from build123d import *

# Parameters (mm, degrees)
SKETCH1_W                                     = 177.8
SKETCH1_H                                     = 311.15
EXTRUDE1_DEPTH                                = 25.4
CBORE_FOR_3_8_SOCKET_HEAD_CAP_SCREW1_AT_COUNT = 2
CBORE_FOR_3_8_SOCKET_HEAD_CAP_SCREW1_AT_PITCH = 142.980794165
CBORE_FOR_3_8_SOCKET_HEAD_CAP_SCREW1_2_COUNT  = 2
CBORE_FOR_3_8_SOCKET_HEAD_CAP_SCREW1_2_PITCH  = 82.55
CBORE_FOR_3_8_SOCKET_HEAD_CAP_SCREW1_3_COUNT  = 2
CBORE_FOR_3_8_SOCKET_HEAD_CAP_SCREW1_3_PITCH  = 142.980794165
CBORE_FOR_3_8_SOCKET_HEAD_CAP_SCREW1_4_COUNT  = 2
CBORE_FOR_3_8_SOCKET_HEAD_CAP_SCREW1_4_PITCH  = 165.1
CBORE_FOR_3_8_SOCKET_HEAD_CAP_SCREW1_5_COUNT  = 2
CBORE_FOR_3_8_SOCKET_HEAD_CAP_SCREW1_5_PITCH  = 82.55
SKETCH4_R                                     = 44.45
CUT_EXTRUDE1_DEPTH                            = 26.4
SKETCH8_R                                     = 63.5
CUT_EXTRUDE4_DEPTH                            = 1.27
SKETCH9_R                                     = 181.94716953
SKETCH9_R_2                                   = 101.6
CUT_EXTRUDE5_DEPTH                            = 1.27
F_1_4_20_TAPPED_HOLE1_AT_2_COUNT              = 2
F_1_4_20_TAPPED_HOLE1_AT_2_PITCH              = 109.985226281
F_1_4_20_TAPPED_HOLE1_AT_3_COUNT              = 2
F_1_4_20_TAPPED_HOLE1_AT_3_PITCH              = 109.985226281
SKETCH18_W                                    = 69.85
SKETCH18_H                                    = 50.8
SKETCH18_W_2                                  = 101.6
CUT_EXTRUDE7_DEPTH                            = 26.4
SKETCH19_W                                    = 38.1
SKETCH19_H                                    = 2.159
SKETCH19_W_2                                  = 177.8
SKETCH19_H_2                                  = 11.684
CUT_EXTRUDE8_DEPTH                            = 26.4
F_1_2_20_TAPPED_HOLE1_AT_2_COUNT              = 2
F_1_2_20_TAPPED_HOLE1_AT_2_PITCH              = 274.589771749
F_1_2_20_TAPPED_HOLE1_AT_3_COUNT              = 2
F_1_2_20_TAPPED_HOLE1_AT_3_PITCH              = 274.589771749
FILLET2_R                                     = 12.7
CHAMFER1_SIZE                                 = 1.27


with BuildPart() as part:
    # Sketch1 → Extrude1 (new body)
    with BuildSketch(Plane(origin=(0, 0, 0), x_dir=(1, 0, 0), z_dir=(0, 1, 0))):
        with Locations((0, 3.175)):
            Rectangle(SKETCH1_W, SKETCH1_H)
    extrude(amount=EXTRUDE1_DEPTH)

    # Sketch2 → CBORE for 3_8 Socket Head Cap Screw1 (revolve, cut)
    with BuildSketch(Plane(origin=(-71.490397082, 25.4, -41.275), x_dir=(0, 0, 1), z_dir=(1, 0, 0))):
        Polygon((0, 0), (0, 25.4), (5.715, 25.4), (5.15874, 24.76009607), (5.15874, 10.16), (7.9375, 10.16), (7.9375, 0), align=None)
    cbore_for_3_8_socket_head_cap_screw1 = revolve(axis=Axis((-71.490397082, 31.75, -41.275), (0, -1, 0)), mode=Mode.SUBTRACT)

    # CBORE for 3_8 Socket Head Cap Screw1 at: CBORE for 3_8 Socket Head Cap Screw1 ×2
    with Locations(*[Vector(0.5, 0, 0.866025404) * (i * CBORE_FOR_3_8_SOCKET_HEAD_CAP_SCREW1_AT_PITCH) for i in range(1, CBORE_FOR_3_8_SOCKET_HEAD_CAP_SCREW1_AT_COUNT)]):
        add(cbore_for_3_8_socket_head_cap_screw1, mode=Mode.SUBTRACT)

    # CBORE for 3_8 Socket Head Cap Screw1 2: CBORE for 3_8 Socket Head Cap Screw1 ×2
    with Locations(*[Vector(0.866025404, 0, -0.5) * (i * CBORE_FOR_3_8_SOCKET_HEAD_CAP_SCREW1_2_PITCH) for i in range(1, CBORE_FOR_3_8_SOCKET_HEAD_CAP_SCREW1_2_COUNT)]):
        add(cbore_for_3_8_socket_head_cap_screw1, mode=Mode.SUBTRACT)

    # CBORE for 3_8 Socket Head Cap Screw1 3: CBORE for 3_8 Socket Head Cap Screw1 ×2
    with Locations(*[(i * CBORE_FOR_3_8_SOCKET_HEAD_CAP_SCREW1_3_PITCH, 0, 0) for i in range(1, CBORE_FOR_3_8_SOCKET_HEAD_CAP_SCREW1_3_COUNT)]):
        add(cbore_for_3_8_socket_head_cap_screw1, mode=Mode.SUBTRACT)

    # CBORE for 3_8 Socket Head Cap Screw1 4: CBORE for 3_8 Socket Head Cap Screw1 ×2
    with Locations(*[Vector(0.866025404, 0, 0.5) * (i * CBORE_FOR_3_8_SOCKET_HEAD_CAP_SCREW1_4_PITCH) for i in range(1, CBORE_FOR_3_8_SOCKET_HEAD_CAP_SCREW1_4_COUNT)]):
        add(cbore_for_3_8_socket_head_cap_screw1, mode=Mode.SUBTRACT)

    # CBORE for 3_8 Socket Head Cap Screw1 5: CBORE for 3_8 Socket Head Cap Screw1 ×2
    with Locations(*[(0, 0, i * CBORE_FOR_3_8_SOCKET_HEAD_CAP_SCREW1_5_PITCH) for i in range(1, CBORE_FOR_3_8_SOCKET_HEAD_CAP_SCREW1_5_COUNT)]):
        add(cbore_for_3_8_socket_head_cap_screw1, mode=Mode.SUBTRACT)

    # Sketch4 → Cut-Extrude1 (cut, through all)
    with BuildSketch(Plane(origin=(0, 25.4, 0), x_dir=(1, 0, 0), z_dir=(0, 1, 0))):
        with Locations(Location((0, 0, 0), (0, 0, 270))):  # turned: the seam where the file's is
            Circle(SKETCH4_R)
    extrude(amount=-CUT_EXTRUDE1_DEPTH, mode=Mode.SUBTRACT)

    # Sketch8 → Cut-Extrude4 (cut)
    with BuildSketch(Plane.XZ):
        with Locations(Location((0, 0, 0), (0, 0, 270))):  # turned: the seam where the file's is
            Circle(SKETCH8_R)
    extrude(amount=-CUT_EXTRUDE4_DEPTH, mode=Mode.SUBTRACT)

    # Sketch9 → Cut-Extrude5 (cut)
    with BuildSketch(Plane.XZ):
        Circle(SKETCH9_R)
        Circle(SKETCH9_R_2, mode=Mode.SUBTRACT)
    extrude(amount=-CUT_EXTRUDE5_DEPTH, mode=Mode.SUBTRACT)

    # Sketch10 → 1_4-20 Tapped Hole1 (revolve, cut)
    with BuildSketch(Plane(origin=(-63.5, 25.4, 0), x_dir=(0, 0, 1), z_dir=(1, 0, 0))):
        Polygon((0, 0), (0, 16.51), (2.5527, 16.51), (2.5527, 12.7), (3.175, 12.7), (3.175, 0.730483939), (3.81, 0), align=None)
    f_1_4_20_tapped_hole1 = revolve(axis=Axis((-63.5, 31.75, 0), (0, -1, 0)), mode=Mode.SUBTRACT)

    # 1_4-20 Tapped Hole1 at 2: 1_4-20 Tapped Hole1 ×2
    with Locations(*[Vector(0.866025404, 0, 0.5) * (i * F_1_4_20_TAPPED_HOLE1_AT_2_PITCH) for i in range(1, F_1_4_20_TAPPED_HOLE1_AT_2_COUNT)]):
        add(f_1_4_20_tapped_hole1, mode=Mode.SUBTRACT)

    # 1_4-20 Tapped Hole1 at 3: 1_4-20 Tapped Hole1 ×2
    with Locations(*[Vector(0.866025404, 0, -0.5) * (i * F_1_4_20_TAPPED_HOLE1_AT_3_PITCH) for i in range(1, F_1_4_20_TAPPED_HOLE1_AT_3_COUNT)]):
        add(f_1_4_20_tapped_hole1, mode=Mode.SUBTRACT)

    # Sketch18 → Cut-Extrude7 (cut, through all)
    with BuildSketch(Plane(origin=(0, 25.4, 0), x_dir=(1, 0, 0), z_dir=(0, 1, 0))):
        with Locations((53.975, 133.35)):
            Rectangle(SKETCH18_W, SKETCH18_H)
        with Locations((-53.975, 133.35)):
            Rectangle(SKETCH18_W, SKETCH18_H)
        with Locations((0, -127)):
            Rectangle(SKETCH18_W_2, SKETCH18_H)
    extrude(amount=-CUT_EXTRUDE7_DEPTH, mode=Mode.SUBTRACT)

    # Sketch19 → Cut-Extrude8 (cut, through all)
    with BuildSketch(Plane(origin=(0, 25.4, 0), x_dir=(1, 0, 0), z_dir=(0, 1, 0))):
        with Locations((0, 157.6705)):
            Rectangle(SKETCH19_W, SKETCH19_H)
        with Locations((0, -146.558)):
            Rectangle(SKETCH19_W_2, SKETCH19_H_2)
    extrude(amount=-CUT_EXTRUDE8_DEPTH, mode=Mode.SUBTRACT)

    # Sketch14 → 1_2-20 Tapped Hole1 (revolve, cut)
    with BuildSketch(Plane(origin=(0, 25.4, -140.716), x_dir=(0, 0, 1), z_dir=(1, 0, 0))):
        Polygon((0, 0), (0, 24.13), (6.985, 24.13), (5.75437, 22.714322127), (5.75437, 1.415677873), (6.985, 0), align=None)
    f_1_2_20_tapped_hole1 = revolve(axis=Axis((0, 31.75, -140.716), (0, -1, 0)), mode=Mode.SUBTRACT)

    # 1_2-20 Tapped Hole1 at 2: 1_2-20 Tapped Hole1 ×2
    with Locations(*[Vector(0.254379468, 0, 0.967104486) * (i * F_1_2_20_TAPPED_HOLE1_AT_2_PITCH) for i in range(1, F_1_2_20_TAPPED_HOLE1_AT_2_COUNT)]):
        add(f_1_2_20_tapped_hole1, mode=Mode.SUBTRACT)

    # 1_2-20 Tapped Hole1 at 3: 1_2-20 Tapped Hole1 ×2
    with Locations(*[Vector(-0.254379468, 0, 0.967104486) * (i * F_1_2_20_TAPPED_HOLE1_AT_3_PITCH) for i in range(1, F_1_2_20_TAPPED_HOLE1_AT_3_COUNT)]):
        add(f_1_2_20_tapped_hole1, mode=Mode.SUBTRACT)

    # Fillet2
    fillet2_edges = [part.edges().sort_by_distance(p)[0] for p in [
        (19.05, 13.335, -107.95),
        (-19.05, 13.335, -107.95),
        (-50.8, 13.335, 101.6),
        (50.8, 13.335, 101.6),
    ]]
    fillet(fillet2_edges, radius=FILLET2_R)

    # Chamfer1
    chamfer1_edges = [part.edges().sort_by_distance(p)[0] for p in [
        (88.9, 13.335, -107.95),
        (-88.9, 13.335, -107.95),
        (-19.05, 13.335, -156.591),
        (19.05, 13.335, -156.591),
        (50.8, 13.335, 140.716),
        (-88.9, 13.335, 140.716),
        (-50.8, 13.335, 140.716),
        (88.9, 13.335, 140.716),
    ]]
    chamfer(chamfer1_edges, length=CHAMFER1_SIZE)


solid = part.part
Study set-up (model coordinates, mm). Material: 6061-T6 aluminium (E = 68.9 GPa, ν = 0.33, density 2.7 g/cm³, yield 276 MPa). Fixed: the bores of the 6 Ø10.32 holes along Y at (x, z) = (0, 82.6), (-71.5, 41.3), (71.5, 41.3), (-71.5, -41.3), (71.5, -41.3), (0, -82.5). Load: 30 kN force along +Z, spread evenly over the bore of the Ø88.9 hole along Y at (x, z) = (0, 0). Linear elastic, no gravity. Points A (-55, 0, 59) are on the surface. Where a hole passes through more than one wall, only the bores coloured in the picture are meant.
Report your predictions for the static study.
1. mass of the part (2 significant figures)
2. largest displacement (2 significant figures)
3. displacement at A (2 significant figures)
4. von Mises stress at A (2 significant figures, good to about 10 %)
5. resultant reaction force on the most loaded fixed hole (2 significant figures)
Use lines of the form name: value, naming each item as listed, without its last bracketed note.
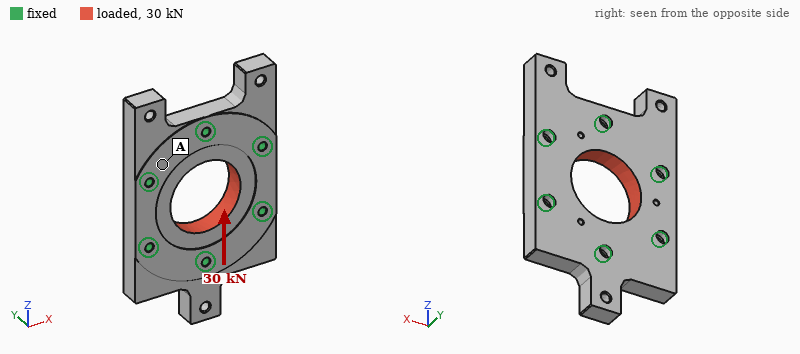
mass of the part: 2.3 kg
largest displacement: 8.2 µm
displacement at A: 1.8 µm
von Mises stress at A: 3.0 MPa
resultant reaction force on the most loaded fixed hole: 6.3 kN
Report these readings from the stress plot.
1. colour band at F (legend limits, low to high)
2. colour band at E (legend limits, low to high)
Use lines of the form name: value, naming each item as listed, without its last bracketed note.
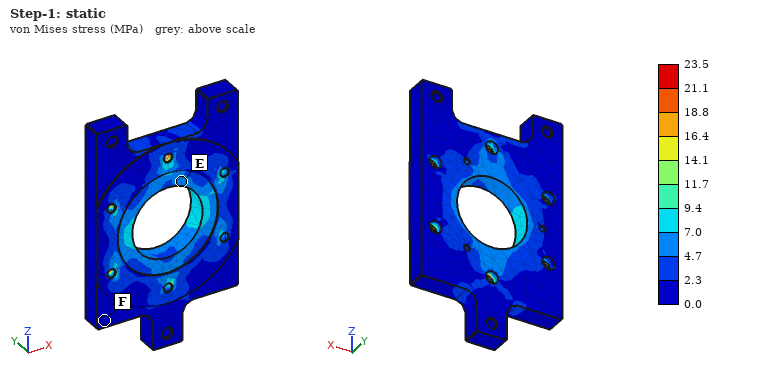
colour band at F: 0.0 to 2.3 MPa
colour band at E: 4.7 to 7.0 MPa
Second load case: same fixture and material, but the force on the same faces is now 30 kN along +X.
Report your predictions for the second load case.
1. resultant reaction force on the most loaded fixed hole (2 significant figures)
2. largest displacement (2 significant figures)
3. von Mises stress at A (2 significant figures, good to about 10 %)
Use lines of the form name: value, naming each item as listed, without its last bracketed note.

resultant reaction force on the most loaded fixed hole: 5.9 kN
largest displacement: 8.5 µm
von Mises stress at A: 2.4 MPa
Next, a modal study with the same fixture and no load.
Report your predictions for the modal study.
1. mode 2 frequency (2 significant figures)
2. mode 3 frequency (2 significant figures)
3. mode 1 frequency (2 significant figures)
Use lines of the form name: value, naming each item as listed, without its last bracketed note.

mode 2 frequency: 2600 Hz
mode 3 frequency: 3400 Hz
mode 1 frequency: 2600 Hz
